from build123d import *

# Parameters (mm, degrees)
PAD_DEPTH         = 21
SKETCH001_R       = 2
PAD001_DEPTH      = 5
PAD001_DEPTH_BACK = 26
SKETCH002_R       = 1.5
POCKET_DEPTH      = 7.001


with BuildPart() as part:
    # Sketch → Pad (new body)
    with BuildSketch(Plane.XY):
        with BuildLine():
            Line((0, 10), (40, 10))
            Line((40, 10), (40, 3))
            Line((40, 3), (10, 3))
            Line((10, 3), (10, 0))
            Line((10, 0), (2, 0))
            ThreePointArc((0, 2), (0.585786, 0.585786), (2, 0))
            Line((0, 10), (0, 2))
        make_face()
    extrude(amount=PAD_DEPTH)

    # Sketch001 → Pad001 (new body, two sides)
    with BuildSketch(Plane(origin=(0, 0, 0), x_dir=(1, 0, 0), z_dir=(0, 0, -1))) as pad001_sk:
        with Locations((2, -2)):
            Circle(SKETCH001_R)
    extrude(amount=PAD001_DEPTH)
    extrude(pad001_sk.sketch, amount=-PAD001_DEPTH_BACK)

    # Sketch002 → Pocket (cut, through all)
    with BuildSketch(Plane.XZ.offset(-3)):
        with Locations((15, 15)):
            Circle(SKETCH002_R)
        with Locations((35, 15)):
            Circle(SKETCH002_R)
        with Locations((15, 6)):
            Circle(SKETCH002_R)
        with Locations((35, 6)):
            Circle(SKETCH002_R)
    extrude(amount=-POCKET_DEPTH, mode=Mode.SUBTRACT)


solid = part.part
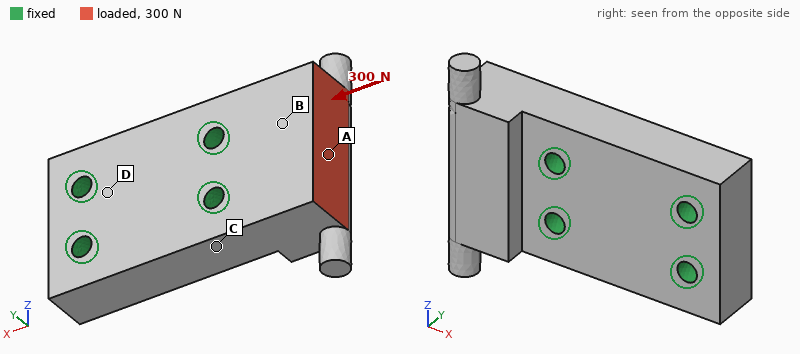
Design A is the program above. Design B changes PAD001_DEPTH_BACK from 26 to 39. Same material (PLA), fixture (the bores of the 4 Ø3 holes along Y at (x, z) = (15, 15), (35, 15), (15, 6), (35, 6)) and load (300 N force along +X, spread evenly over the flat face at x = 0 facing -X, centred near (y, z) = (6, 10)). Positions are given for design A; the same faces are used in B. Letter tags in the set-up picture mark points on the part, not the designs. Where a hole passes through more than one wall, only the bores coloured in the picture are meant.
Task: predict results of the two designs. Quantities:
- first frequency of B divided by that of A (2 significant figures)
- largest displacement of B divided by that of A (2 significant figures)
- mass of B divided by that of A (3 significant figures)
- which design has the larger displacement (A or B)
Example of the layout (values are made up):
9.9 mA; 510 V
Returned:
0.40; 1.3; 1.03; B
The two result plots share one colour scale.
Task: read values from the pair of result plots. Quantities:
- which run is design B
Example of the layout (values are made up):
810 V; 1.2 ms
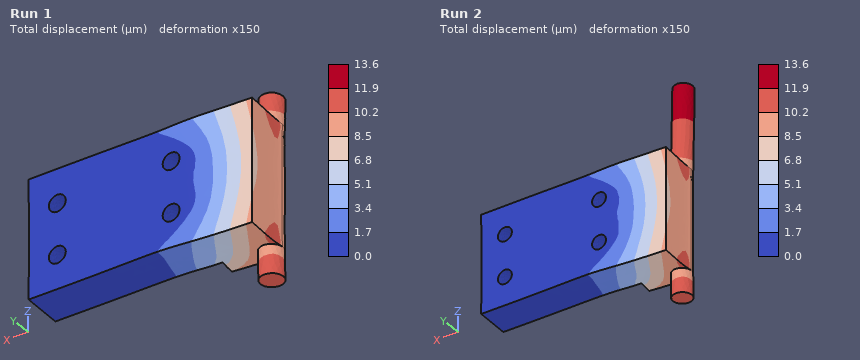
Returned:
Run 2
